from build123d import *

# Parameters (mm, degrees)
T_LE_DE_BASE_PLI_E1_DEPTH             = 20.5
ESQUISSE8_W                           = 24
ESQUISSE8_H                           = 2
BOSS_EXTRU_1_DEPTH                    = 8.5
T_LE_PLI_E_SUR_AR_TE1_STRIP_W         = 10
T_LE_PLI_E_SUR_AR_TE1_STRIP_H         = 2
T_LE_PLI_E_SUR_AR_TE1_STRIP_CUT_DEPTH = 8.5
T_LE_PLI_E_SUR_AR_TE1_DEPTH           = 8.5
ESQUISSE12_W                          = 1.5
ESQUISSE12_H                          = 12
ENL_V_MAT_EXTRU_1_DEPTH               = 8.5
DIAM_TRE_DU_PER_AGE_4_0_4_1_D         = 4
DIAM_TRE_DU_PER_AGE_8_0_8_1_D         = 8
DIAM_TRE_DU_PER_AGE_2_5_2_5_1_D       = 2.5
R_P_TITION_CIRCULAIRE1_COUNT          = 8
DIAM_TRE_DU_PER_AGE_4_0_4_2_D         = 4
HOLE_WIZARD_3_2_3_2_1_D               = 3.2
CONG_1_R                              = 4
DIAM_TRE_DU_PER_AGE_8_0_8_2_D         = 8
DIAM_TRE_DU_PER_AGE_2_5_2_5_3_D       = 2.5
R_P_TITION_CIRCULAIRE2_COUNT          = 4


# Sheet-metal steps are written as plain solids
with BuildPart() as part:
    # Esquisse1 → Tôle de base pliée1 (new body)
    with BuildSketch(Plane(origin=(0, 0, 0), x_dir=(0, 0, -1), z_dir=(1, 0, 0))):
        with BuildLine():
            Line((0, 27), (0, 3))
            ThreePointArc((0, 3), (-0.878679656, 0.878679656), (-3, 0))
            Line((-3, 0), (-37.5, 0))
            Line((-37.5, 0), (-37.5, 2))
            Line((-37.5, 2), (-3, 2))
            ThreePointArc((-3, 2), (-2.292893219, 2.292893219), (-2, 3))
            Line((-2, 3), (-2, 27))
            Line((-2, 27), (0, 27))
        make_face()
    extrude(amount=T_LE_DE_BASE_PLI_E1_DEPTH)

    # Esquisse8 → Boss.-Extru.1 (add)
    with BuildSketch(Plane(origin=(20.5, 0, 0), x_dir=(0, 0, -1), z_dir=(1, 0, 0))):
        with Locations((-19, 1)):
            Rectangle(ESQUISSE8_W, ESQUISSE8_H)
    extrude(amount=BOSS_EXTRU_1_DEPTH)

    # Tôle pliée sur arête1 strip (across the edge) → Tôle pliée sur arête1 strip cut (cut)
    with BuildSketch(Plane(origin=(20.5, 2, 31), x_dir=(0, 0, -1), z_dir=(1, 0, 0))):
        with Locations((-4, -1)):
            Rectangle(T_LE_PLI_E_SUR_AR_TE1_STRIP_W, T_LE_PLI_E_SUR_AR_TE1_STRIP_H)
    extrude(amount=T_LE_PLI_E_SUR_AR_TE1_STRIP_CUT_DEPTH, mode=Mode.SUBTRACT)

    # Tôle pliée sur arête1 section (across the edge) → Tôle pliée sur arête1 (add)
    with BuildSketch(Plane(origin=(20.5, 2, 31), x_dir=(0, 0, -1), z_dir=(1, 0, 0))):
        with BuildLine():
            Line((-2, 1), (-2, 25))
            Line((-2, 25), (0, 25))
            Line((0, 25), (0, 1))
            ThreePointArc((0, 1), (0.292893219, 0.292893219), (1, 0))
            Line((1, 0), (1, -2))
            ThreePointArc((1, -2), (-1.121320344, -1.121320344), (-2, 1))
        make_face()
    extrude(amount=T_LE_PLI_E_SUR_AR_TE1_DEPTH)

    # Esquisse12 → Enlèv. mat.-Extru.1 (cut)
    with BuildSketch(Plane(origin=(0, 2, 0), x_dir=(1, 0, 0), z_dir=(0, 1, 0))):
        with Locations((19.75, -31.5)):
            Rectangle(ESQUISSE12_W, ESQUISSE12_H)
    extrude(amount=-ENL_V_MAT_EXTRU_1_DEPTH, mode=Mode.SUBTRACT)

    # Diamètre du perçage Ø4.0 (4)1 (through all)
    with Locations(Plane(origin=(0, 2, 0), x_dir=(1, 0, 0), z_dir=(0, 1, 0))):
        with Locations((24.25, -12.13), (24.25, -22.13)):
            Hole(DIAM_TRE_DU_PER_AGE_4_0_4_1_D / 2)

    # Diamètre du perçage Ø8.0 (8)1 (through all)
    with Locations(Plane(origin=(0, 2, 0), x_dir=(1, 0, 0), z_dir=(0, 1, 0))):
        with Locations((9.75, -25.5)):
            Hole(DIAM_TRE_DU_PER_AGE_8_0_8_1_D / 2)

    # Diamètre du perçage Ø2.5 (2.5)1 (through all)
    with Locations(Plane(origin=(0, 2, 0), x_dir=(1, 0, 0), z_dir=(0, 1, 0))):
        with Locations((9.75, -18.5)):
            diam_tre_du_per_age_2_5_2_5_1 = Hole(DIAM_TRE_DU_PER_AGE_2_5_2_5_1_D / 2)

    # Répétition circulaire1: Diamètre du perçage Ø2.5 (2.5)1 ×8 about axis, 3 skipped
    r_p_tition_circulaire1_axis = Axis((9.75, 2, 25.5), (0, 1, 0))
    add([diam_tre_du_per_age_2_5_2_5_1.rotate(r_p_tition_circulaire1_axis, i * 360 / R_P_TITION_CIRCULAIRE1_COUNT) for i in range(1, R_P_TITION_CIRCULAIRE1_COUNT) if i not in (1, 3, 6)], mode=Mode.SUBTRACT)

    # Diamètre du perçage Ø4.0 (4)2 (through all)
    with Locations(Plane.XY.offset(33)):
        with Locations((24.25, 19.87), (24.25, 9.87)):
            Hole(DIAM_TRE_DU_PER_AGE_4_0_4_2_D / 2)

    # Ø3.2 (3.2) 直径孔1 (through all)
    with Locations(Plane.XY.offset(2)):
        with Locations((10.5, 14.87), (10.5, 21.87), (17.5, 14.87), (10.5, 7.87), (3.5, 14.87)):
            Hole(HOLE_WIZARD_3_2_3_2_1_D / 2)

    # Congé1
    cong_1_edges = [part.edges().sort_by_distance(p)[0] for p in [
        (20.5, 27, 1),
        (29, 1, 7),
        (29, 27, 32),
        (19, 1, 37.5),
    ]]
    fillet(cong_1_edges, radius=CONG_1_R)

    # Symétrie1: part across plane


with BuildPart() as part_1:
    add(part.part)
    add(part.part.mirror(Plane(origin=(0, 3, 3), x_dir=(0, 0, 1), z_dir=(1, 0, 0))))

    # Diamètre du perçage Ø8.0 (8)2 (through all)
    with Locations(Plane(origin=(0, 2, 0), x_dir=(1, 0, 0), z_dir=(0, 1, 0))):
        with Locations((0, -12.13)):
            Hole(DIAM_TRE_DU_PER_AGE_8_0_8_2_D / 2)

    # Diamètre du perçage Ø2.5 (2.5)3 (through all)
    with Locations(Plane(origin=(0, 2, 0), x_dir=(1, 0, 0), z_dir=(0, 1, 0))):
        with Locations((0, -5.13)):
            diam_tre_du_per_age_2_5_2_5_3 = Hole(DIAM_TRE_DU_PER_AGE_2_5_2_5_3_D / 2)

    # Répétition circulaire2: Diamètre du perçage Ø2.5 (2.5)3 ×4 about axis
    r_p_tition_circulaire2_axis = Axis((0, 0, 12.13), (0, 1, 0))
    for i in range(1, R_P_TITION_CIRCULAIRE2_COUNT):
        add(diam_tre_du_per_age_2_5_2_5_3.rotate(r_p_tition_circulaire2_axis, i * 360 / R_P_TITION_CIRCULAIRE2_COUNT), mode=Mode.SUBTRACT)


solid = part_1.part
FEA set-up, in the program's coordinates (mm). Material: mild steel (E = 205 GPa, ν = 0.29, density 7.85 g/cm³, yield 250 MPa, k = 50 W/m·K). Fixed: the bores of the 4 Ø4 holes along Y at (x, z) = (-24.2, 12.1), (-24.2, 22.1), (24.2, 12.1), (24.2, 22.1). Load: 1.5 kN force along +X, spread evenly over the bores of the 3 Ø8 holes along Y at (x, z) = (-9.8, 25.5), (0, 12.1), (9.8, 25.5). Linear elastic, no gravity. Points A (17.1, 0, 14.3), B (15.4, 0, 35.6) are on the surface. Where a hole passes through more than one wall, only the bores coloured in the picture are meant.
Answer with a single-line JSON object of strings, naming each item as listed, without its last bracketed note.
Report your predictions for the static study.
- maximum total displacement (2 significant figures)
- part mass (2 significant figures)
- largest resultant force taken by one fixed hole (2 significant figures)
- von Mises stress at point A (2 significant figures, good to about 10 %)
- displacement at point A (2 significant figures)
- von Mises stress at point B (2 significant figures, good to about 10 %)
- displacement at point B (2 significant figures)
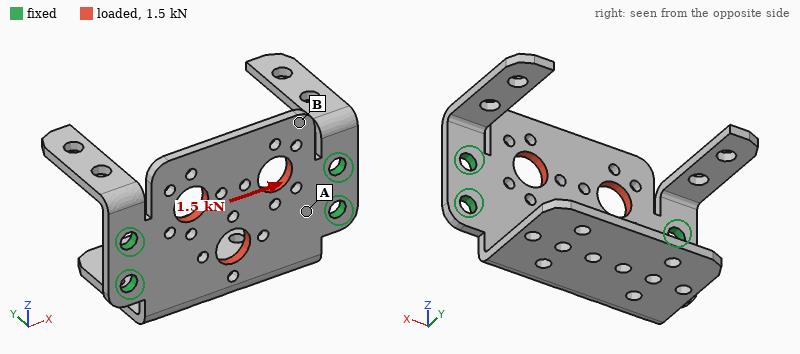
{"maximum total displacement": "3.6 µm", "part mass": "46 g", "largest resultant force taken by one fixed hole": "390 N", "von Mises stress at point A": "19 MPa", "displacement at point A": "0.61 µm", "von Mises stress at point B": "6.9 MPa", "displacement at point B": "3.3 µm"}
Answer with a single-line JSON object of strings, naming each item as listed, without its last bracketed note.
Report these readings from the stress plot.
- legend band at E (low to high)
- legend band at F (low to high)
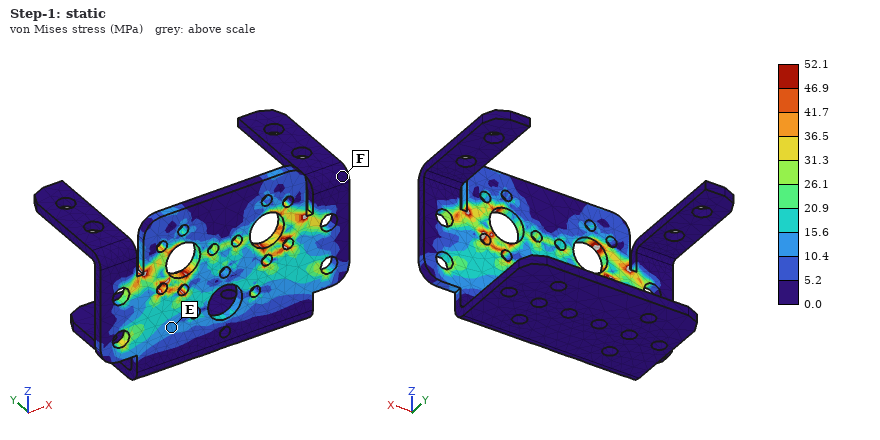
{"legend band at E": "10.4 to 15.6 MPa", "legend band at F": "0.0 to 5.2 MPa"}
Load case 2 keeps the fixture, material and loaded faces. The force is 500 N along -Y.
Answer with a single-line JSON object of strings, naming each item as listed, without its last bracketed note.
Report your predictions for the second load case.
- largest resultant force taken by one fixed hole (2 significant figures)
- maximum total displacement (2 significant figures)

{"largest resultant force taken by one fixed hole": "200 N", "maximum total displacement": "0.10 mm"}
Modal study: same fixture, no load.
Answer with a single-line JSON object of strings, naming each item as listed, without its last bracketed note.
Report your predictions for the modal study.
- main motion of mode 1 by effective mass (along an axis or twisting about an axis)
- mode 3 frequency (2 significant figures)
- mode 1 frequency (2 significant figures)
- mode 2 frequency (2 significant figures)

{"main motion of mode 1 by effective mass": "along Z", "mode 3 frequency": "1700 Hz", "mode 1 frequency": "1400 Hz", "mode 2 frequency": "1700 Hz"}
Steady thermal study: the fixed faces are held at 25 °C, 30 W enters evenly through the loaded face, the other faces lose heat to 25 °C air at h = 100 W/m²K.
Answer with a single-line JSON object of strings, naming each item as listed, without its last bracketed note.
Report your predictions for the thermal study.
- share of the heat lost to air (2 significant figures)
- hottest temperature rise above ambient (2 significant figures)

{"share of the heat lost to air": "54 %", "hottest temperature rise above ambient": "79 K"}
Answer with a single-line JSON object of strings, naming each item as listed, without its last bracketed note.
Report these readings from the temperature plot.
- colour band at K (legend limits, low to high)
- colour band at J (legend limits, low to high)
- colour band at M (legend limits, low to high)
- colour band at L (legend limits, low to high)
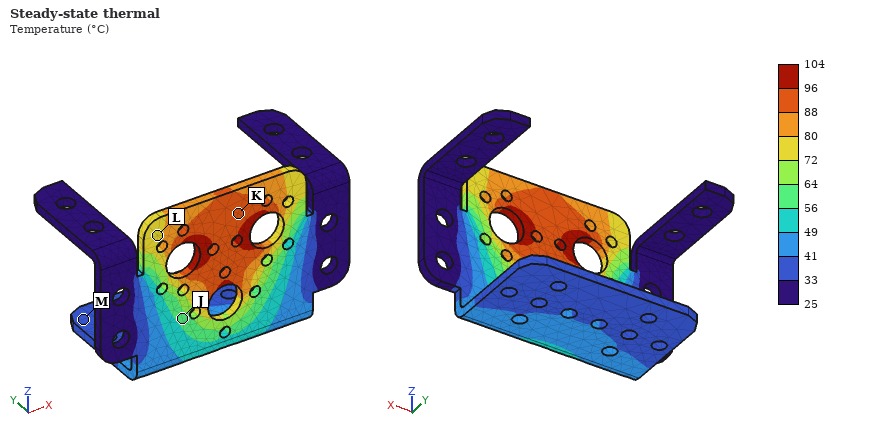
{"colour band at K": "88 to 96 °C", "colour band at J": "56 to 64 °C", "colour band at M": "33 to 41 °C", "colour band at L": "72 to 80 °C"}
